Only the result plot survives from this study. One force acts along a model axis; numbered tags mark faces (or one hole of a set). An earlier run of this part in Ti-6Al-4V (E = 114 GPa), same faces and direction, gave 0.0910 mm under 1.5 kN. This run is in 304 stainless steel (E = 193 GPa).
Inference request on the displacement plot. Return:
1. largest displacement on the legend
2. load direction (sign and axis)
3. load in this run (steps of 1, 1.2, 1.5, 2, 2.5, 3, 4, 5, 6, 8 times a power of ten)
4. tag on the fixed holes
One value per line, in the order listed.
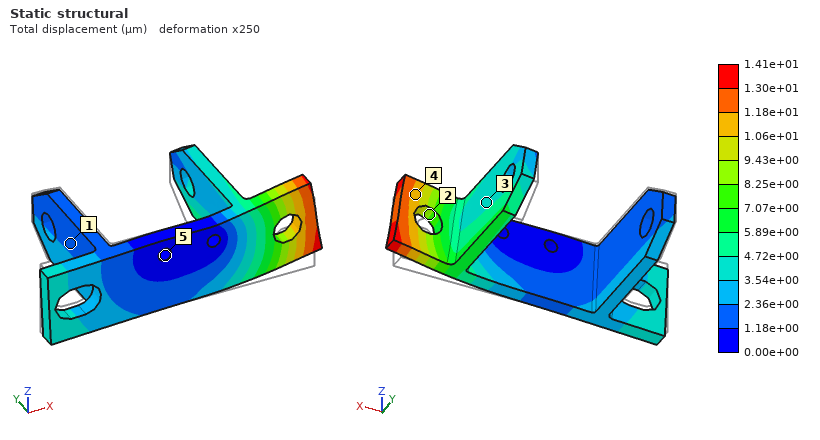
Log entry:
1.41e+01 µm
+Z
400 N
5
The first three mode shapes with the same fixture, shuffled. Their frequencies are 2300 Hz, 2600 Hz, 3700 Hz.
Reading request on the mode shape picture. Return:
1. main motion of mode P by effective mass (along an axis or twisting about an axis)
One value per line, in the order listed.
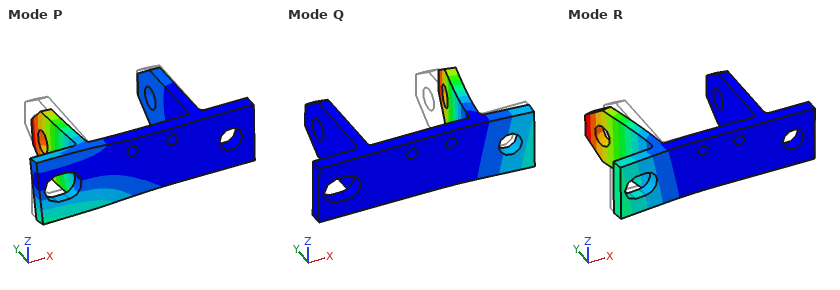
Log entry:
along Z
